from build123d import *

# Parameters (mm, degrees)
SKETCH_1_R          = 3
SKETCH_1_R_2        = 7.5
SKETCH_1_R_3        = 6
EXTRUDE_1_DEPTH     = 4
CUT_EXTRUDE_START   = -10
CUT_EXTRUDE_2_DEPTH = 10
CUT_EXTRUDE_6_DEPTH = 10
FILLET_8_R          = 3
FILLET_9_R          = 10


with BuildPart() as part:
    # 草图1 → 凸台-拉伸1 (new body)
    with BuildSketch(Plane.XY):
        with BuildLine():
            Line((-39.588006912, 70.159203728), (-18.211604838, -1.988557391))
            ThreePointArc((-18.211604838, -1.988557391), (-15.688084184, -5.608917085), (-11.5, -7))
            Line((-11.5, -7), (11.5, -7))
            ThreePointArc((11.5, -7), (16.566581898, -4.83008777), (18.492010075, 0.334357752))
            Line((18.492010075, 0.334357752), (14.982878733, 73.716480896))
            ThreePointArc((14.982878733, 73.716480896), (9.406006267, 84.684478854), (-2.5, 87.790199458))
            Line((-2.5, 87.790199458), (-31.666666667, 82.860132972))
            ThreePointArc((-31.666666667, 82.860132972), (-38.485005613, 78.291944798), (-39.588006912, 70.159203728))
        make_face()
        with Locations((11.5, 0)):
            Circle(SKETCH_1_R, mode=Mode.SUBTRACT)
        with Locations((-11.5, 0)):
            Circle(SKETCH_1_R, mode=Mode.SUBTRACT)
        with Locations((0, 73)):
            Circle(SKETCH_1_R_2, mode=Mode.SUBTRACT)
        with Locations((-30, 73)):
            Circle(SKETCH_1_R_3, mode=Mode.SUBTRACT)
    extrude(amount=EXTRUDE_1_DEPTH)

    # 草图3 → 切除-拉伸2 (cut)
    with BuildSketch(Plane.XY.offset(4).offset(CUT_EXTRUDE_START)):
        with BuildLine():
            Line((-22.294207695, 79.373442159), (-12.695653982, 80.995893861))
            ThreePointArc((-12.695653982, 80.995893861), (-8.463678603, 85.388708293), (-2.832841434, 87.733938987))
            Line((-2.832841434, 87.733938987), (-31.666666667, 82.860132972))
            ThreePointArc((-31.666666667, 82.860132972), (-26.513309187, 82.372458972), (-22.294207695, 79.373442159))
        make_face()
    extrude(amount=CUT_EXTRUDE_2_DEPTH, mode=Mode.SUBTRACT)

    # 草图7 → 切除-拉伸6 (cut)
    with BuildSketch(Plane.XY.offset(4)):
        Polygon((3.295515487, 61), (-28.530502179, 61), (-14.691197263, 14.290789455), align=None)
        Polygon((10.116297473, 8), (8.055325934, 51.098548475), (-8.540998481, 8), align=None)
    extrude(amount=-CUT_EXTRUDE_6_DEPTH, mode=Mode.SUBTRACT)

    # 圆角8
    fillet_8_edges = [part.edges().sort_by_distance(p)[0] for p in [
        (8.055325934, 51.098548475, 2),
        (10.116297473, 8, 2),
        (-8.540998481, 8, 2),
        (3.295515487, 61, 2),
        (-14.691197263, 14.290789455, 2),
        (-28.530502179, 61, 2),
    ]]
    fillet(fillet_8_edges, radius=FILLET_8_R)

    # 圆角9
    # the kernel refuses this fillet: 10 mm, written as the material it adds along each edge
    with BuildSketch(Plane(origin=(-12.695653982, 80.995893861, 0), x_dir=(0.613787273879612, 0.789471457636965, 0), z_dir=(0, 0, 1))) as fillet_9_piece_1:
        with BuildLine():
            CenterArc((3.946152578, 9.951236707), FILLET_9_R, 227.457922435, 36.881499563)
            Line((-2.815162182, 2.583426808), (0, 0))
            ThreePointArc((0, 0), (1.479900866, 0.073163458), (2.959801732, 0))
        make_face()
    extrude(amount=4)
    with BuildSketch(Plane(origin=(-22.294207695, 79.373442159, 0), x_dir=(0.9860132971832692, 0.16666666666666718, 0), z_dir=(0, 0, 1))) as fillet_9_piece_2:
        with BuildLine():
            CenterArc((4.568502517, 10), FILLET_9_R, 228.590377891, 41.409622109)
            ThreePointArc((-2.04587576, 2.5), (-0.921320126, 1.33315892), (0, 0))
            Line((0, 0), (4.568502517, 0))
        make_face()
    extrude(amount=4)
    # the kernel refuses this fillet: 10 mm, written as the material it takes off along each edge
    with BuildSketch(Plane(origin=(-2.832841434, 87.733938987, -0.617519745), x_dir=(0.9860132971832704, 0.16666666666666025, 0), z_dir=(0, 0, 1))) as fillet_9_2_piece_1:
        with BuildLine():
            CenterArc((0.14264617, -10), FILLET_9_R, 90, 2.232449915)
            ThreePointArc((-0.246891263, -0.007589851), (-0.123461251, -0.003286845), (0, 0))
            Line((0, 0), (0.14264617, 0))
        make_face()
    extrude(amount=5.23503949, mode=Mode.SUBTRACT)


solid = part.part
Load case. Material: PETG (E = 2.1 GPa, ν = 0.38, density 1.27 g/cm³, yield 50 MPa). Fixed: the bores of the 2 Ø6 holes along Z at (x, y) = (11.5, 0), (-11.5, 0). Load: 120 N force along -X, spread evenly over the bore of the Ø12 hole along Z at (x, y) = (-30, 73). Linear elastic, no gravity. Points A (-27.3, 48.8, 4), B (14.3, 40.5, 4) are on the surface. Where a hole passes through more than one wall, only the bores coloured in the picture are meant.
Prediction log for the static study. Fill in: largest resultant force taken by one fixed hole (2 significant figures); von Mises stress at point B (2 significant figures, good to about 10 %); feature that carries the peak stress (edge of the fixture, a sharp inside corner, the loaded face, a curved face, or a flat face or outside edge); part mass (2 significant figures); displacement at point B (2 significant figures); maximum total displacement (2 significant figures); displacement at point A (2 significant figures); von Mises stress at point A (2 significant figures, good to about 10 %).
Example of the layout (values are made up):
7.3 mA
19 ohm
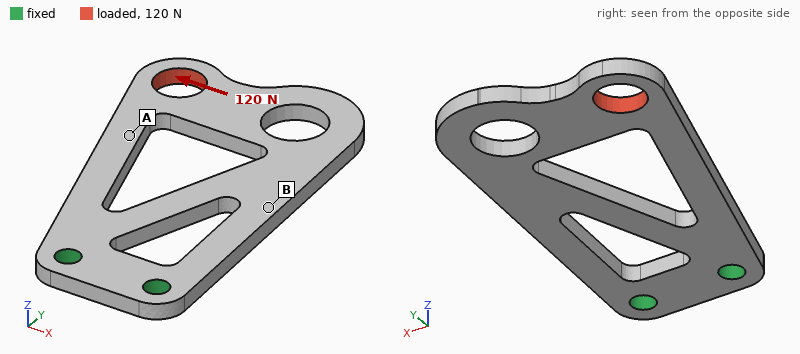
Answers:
310 N
6.1 MPa
edge of the fixture
14 g
0.49 mm
1.1 mm
0.68 mm
2.3 MPa
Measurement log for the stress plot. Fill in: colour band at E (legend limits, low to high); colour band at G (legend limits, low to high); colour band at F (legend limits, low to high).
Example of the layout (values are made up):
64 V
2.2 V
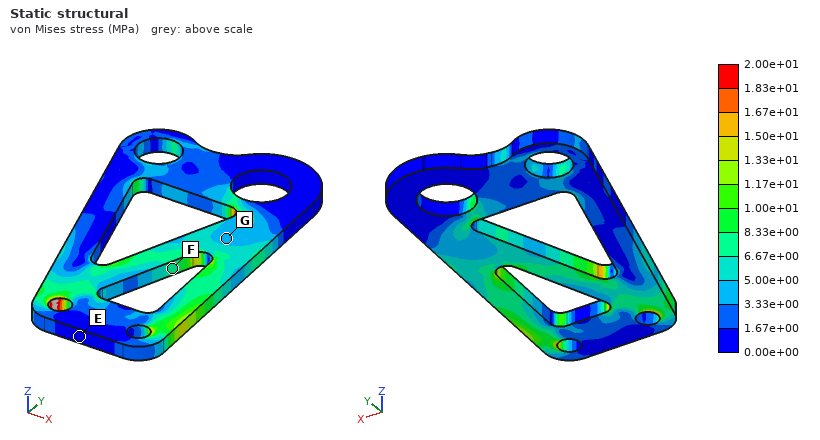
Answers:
0.00e+00 to 1.67e+00 MPa
3.33e+00 to 5.00e+00 MPa
6.67e+00 to 8.33e+00 MPa
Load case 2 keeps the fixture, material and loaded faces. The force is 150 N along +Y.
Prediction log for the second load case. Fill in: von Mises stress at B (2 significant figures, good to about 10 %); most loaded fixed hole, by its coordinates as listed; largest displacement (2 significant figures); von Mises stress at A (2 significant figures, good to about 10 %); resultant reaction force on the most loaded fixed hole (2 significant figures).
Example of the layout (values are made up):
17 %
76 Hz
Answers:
1.9 MPa
(-11.5, 0)
0.53 mm
5.2 MPa
240 N
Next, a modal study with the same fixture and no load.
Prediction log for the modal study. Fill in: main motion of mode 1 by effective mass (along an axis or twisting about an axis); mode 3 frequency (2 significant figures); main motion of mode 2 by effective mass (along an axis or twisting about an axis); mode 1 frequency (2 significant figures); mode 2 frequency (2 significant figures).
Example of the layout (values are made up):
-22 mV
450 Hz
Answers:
along Z
670 Hz
twisting about Y
100 Hz
290 Hz
